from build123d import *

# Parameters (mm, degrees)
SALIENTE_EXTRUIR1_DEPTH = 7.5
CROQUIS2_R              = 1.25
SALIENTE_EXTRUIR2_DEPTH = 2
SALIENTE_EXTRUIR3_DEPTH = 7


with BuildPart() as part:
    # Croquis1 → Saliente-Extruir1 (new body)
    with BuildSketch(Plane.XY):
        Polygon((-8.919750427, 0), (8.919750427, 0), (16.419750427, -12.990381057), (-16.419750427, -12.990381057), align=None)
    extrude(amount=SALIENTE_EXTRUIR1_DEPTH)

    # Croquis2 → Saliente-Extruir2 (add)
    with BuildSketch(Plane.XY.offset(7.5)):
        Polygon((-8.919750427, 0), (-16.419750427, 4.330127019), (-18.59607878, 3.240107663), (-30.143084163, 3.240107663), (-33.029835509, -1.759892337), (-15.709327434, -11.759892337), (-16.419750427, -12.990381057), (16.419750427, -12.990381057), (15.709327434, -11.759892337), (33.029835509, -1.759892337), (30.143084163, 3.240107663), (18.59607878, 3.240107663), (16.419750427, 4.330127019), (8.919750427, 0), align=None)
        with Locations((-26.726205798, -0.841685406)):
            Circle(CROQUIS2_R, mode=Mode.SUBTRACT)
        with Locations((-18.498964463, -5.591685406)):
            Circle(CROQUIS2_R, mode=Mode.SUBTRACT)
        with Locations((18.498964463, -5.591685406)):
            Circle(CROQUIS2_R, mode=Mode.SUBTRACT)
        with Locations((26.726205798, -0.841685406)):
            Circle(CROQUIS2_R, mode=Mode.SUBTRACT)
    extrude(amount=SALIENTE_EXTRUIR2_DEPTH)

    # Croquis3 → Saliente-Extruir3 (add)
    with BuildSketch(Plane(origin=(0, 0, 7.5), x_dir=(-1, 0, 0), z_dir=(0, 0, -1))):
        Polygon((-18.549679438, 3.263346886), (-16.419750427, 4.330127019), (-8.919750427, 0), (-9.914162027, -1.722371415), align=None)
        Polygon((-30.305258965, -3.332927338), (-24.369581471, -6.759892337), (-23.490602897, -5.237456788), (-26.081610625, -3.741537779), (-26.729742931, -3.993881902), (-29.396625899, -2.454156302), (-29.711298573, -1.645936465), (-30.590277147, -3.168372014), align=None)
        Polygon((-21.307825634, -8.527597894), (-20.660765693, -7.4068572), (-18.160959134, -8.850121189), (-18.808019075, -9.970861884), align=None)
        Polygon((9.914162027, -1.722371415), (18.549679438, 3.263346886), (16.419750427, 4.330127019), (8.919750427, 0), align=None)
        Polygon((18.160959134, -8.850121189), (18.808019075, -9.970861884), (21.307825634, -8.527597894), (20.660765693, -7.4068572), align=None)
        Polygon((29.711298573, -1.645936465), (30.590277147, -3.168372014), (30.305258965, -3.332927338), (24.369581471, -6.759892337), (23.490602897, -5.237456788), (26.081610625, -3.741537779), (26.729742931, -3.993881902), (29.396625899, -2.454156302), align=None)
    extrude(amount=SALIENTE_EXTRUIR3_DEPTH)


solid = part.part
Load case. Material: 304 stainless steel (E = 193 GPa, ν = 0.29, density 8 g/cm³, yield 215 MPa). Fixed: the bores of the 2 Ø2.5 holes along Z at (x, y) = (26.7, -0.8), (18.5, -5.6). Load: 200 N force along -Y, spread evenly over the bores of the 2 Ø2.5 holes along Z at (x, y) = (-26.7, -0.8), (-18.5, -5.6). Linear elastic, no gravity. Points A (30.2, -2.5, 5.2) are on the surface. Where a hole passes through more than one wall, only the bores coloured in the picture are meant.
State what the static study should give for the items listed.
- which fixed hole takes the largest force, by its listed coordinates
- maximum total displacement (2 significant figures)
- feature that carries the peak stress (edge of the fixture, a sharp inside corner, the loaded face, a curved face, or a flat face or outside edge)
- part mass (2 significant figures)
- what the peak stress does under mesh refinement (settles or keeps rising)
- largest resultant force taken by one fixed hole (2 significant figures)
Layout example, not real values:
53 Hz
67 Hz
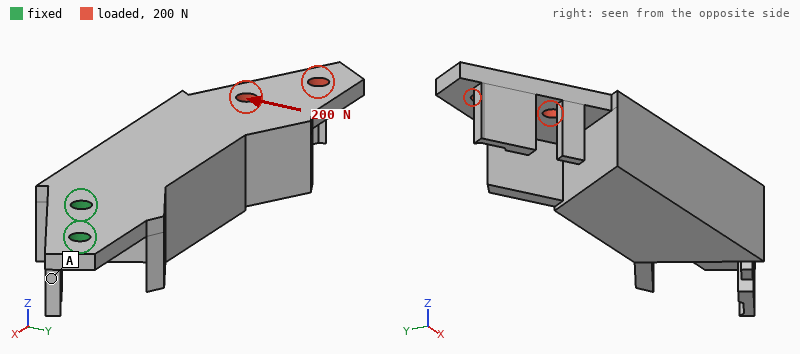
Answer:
(18.5, -5.6)
86 µm
a sharp inside corner
35 g
keeps rising
840 N
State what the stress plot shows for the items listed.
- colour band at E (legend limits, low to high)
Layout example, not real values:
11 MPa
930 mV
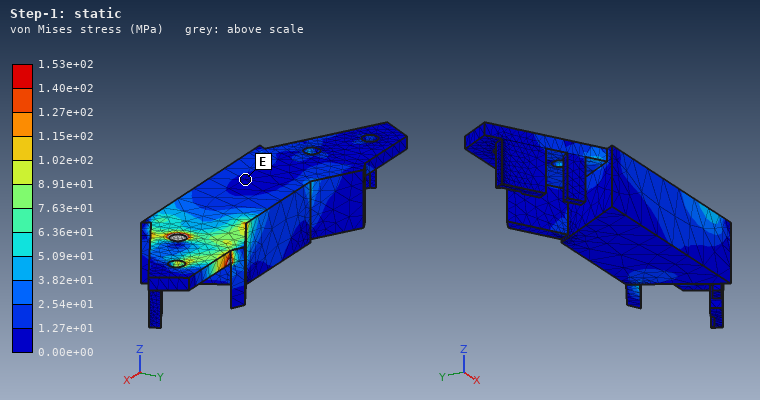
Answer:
0.00e+00 to 1.27e+01 MPa
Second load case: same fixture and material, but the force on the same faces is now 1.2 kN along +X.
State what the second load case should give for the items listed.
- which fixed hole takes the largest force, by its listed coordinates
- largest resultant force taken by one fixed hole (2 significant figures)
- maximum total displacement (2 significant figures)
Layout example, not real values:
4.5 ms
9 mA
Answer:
(18.5, -5.6)
820 N
48 µm
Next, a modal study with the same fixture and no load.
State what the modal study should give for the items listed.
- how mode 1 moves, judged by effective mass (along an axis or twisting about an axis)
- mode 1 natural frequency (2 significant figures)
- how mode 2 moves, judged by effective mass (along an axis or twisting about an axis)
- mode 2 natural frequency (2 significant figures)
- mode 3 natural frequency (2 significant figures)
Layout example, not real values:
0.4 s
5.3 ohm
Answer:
along Z
820 Hz
along Y
2800 Hz
4600 Hz
